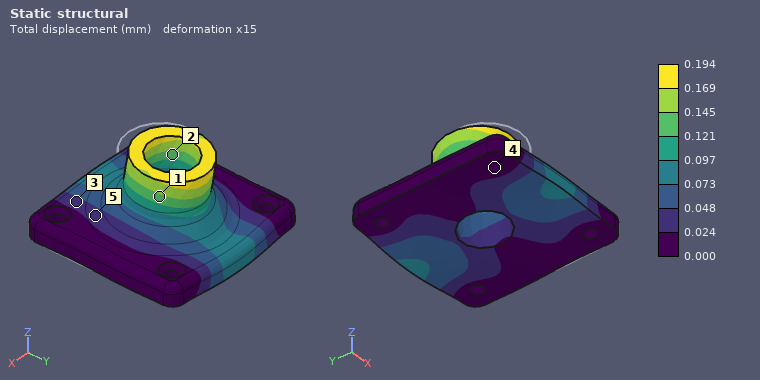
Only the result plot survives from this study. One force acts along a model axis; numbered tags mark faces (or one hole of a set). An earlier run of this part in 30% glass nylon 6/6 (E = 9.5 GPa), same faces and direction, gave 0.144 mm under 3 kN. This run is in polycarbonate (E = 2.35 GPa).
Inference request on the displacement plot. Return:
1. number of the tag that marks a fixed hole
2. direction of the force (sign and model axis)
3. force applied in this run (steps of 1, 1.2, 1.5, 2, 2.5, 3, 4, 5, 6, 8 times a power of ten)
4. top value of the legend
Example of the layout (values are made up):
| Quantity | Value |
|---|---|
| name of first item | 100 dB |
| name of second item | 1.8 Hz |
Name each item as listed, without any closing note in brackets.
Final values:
| Quantity | Value |
|---|---|
| number of the tag that marks a fixed hole | 4 |
| direction of the force | +Y |
| force applied in this run | 1 kN |
| top value of the legend | 0.194 mm |
